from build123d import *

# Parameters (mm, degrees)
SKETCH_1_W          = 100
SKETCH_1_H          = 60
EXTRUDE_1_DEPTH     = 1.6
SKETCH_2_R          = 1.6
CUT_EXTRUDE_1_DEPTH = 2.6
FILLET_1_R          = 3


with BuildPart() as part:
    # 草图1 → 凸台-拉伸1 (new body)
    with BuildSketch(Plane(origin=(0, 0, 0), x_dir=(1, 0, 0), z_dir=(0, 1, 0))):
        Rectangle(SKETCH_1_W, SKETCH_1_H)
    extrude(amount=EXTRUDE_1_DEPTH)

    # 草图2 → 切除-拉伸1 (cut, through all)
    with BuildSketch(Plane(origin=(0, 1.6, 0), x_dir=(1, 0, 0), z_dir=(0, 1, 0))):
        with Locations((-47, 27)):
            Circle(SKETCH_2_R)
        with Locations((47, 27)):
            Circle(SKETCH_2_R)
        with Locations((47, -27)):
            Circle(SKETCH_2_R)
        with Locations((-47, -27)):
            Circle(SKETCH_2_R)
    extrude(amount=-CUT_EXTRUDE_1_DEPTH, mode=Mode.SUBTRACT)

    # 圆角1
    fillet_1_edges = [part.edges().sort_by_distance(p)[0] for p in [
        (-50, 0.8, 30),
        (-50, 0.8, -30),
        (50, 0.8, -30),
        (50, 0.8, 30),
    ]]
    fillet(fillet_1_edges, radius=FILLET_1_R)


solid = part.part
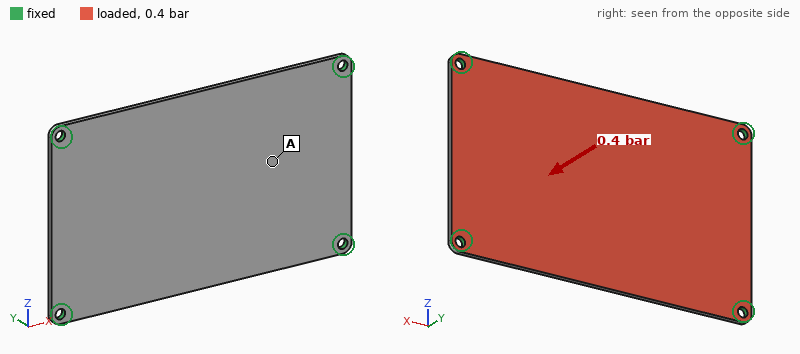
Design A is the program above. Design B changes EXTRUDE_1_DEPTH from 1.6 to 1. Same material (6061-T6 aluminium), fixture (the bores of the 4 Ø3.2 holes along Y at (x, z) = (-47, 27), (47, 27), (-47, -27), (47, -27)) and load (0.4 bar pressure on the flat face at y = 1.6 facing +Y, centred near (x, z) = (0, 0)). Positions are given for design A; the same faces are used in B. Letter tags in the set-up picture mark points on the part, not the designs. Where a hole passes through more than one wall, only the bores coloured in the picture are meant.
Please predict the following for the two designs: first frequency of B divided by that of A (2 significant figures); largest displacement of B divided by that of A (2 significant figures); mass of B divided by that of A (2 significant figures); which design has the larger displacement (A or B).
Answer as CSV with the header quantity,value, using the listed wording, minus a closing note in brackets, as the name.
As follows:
quantity,value
first frequency of B divided by that of A,0.63
largest displacement of B divided by that of A,4.0
mass of B divided by that of A,0.62
which design has the larger displacement,B
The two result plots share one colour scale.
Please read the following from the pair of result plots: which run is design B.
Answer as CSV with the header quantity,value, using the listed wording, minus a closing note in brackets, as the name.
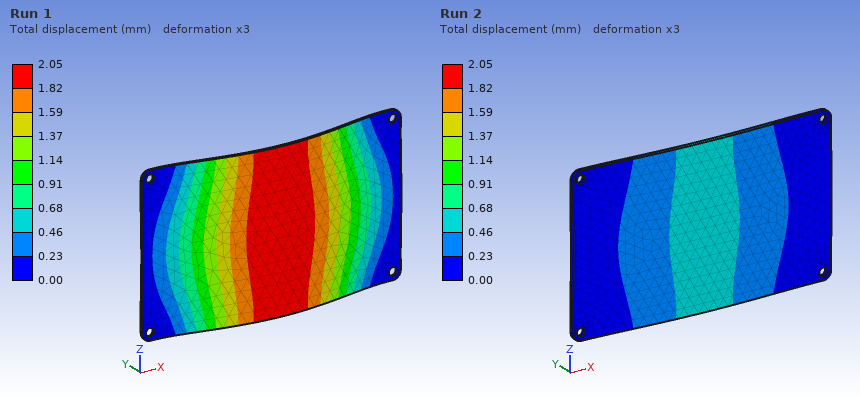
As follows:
quantity,value
which run is design B,Run 1
